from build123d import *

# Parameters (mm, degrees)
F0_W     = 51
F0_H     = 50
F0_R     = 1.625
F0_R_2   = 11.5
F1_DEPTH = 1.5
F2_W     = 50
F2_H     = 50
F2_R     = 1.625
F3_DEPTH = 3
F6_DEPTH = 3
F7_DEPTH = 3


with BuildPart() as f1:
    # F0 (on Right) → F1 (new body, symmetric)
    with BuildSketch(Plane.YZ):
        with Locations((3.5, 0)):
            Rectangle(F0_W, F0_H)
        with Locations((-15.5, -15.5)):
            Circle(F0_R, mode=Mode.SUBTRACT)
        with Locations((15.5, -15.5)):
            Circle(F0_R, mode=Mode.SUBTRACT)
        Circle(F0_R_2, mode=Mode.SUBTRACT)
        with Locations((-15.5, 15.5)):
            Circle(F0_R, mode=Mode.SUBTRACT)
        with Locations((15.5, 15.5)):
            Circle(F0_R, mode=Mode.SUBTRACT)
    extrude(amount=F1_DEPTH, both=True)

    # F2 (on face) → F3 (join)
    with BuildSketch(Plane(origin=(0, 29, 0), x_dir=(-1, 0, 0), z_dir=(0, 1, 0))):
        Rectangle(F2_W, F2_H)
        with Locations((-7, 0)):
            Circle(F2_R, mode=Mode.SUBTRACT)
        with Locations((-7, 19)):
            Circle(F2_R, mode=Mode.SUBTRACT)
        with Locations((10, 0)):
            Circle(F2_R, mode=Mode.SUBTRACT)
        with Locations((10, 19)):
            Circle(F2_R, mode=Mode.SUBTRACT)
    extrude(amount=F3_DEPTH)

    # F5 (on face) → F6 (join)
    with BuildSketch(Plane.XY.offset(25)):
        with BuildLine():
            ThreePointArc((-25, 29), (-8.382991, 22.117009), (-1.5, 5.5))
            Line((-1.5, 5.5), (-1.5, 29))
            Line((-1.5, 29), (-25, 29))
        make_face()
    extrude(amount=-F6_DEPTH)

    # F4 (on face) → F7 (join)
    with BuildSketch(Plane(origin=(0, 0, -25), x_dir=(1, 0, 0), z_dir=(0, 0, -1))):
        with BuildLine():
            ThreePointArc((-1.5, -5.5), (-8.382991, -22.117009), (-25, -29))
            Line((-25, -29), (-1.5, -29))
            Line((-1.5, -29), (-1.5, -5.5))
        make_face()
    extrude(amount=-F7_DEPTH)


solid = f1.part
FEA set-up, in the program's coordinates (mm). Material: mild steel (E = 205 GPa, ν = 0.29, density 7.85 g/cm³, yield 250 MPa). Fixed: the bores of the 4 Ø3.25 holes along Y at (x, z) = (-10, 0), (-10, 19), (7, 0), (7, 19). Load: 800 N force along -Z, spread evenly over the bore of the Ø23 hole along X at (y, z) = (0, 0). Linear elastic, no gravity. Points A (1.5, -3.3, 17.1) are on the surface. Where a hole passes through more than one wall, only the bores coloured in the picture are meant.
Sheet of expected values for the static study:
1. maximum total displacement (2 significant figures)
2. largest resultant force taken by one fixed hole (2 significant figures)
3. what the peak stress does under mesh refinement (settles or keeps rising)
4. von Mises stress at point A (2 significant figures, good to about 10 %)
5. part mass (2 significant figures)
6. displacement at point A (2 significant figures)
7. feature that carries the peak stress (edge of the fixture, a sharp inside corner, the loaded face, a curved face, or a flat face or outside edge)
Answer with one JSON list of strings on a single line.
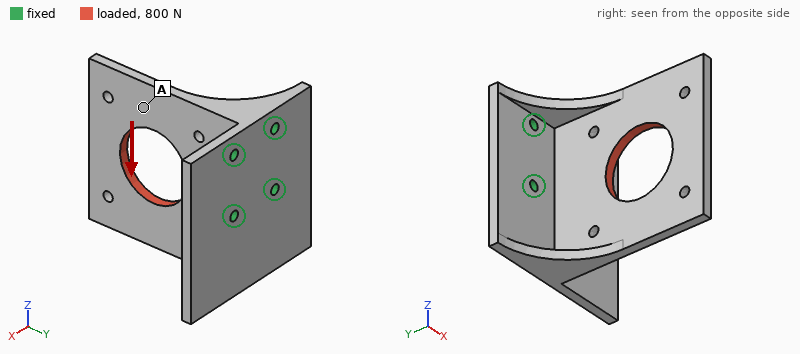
["42 µm", "710 N", "keeps rising", "13 MPa", "110 g", "25 µm", "edge of the fixture"]
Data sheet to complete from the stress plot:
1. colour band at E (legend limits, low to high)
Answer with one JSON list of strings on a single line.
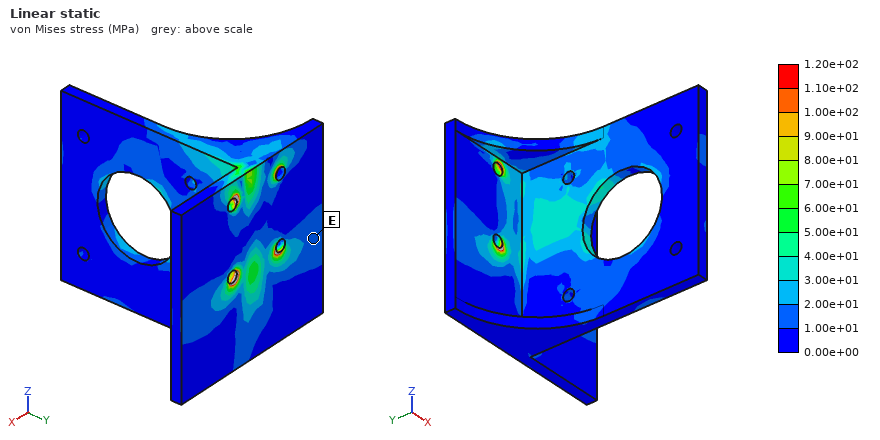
["1.00e+01 to 2.00e+01 MPa"]
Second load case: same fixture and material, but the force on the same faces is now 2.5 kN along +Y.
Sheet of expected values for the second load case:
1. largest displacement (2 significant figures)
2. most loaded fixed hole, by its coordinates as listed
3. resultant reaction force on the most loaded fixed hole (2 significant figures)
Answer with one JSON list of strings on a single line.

["38 µm", "(7, 0)", "1.4 kN"]
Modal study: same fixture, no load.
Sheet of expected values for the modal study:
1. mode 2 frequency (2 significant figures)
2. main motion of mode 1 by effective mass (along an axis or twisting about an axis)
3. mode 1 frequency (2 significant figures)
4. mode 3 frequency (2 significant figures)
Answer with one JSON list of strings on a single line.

["2500 Hz", "along X", "1100 Hz", "3700 Hz"]
